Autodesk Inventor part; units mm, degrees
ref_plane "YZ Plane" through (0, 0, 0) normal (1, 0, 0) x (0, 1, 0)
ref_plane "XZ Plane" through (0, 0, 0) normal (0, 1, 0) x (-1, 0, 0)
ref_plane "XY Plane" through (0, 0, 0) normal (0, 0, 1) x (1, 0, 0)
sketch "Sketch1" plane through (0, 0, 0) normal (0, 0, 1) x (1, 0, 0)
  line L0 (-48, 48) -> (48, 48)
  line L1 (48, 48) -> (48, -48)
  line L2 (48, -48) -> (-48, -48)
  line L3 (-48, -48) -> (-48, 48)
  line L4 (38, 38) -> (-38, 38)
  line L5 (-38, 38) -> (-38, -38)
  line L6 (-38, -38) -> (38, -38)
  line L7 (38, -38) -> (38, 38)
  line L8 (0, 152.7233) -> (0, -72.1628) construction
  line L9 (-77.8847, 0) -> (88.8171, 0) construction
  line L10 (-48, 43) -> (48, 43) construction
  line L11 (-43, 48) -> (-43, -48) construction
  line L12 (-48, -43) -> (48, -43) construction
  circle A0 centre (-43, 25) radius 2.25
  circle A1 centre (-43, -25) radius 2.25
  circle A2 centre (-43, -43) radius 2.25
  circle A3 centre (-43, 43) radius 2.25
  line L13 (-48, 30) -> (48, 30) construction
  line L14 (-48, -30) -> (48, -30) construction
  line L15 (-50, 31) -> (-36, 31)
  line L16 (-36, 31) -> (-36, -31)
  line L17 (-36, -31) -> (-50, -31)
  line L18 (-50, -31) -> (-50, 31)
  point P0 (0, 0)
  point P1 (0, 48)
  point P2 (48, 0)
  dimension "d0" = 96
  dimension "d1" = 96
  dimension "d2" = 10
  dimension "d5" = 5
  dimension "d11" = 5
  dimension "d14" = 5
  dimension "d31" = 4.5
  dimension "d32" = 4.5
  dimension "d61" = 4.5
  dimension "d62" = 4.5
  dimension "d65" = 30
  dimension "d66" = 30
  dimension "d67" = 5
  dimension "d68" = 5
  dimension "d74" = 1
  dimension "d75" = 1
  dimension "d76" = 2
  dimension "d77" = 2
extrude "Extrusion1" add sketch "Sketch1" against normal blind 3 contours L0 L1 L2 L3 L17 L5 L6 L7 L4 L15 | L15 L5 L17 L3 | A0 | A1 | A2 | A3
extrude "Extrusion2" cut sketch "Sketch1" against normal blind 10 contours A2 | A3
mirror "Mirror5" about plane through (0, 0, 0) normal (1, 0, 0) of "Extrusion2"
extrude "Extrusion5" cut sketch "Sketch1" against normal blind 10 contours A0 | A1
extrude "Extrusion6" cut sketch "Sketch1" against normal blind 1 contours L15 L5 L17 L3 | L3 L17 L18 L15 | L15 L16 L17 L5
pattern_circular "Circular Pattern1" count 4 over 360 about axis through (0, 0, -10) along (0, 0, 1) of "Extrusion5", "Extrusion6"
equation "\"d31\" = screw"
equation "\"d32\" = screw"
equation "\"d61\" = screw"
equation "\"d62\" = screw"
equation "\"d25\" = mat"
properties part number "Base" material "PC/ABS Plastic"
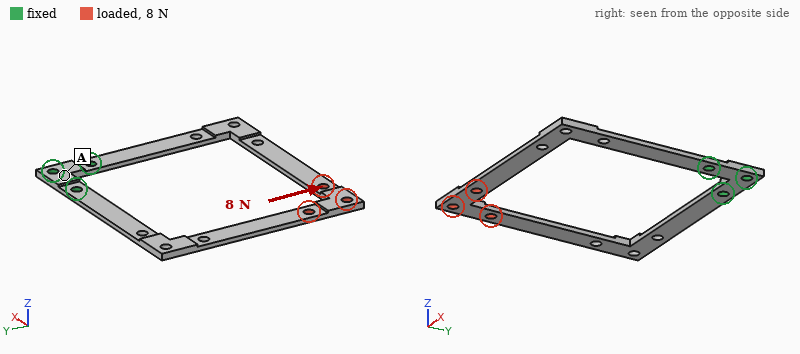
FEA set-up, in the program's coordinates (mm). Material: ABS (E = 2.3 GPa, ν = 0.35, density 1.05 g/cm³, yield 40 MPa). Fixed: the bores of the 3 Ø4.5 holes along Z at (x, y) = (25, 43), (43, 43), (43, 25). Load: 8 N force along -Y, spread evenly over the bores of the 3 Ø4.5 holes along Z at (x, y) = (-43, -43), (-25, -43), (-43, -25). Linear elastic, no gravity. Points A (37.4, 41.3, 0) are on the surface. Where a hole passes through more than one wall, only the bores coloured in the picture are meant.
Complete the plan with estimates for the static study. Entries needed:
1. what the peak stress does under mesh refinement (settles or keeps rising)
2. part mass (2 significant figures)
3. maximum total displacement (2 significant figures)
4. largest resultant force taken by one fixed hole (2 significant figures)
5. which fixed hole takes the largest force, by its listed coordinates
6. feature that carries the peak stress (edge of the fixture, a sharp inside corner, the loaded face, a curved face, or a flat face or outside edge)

keeps rising
7.8 g
1.4 mm
12 N
(25, 43)
edge of the fixture
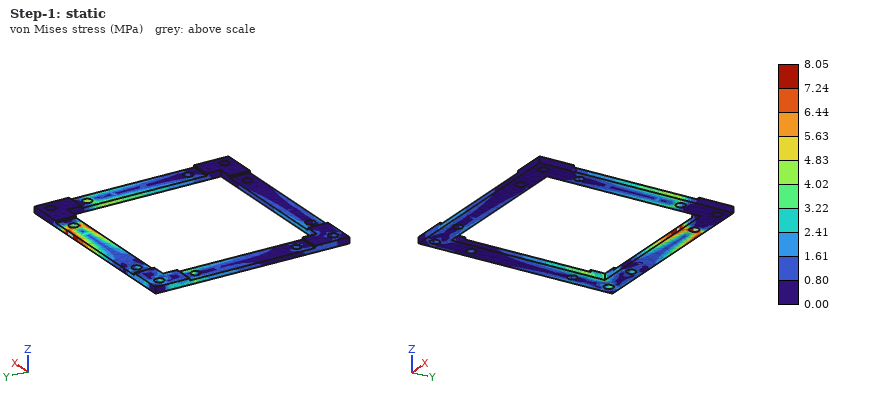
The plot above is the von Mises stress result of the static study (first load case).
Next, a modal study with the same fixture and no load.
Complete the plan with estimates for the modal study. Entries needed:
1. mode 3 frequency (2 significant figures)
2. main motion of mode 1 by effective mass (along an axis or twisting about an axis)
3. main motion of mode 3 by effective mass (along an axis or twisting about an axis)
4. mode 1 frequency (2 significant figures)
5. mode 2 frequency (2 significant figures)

120 Hz
along Z
along Z
29 Hz
63 Hz
